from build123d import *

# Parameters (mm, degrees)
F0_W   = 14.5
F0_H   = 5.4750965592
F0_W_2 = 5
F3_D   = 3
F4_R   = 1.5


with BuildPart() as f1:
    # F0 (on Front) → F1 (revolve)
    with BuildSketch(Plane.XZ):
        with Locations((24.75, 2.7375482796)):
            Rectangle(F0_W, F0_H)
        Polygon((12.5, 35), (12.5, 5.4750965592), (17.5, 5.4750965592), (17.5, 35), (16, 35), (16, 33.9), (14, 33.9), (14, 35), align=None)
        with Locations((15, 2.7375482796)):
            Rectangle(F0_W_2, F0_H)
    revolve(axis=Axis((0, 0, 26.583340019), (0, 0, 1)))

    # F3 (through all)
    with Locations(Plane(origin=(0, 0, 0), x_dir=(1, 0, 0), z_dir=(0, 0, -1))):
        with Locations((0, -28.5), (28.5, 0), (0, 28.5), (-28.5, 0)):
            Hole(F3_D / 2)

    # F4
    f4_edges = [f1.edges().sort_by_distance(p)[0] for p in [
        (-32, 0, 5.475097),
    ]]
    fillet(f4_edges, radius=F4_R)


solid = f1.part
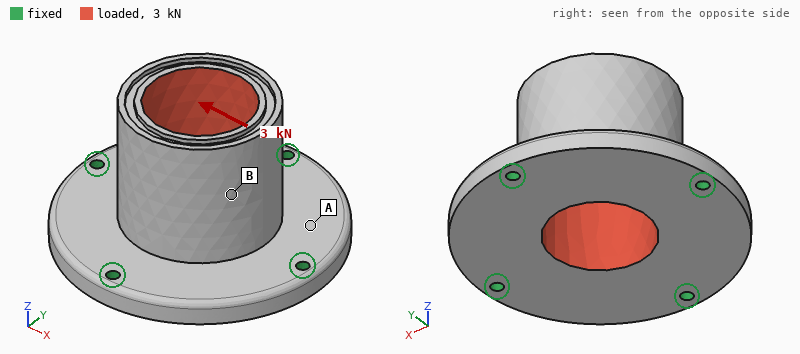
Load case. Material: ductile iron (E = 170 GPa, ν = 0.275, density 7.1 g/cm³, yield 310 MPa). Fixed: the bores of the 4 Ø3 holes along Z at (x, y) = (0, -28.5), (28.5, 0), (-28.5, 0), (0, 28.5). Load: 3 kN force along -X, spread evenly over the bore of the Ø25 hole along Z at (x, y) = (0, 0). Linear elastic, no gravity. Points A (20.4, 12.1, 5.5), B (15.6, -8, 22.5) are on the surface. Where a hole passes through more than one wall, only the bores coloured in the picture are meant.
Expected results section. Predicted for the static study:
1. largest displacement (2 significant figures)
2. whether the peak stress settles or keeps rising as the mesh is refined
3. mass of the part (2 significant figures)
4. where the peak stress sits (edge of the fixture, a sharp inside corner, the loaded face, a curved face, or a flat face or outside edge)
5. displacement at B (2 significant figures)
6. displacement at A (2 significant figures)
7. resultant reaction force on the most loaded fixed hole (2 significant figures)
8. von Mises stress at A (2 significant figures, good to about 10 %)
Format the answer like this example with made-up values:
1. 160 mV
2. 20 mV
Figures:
1. 16 µm
2. keeps rising
3. 200 g
4. edge of the fixture
5. 11 µm
6. 3.8 µm
7. 1.3 kN
8. 18 MPa
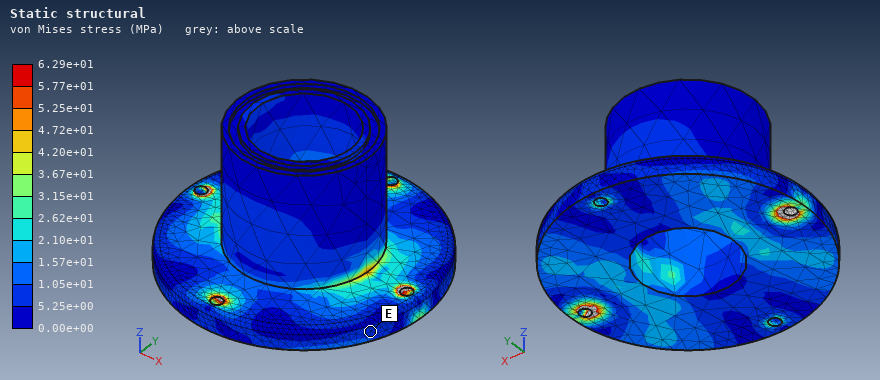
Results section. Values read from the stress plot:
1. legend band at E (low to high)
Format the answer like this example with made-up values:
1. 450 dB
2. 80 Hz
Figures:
1. 5.25e+00 to 1.05e+01 MPa
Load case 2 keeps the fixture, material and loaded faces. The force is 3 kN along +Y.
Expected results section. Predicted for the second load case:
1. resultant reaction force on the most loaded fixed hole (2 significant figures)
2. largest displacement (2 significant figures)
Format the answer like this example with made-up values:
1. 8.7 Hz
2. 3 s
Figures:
1. 1.3 kN
2. 16 µm
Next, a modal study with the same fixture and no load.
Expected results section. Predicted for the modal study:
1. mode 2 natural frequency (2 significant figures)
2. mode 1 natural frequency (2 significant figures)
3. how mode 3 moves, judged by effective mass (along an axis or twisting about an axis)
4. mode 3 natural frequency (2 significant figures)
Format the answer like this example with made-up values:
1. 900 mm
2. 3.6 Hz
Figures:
1. 7100 Hz
2. 7100 Hz
3. along Z
4. 8600 Hz
